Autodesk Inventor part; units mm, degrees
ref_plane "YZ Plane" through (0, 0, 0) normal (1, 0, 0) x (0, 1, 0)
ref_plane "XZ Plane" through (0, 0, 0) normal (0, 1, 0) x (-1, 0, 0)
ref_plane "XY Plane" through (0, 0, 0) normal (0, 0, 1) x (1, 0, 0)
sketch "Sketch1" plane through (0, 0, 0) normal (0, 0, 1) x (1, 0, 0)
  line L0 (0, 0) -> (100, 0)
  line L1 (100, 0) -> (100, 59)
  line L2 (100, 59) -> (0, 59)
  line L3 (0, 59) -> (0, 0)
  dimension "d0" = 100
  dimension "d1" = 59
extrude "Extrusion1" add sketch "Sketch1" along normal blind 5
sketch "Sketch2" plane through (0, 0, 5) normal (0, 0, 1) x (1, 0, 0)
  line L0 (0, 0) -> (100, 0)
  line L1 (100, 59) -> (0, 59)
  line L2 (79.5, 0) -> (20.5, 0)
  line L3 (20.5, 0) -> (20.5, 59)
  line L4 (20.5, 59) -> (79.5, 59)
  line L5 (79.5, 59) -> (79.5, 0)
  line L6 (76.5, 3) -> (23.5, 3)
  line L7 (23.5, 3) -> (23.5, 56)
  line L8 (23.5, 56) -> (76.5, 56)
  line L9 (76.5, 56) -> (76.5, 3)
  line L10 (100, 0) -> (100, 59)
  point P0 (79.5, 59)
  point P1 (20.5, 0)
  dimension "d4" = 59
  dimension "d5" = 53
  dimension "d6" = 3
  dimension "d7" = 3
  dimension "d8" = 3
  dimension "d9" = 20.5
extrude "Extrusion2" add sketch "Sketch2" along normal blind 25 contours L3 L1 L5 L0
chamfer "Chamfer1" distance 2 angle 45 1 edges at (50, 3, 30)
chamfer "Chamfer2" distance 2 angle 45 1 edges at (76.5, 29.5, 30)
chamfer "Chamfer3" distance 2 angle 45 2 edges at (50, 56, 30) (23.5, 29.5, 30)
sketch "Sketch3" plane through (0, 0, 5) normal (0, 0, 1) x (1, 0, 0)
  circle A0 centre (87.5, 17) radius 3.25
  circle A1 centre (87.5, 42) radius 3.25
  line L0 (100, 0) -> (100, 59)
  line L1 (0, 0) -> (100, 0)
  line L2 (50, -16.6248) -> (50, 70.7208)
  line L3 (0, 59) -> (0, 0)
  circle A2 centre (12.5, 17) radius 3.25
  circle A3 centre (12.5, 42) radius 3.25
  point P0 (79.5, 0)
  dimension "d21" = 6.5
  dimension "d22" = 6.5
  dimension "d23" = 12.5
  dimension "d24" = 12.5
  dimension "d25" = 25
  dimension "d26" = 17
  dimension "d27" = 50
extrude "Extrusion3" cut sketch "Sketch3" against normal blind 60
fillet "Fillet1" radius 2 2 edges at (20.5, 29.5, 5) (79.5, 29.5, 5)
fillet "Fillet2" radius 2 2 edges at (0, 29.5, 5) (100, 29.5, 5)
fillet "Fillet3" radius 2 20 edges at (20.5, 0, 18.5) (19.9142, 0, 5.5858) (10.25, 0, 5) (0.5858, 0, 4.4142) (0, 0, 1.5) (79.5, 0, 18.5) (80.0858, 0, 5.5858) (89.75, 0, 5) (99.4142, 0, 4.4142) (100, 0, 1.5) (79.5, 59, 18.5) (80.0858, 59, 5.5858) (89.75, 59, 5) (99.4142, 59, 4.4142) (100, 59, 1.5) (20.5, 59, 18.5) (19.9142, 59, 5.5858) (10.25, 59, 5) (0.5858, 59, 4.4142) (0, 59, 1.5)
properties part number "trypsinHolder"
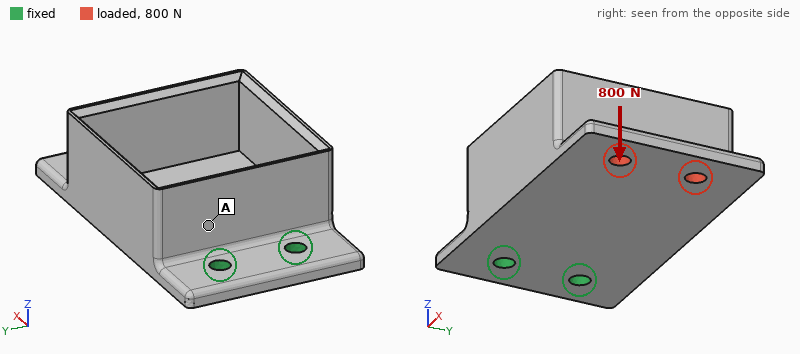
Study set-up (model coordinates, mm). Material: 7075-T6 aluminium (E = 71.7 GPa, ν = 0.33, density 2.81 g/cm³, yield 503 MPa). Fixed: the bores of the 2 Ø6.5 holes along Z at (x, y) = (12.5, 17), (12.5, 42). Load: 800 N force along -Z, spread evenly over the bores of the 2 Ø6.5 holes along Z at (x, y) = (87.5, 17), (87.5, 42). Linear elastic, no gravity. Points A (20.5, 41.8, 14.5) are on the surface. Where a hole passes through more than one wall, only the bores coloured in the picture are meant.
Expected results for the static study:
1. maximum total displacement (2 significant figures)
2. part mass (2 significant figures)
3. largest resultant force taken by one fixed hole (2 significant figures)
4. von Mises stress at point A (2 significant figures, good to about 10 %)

1.4 mm
130 g
470 N
37 MPa
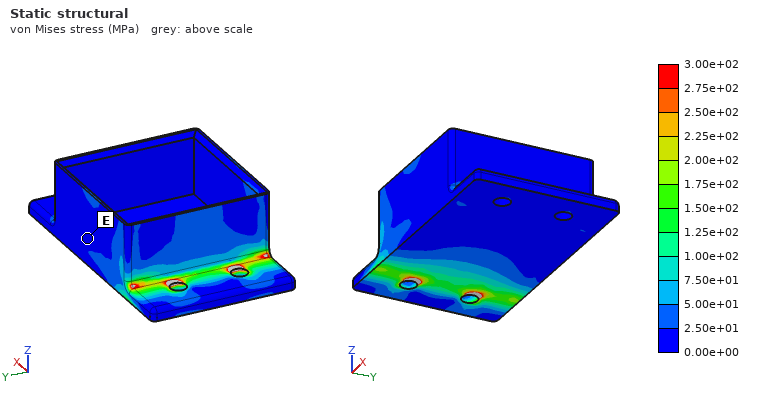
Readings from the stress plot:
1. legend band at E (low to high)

0.00e+00 to 2.50e+01 MPa
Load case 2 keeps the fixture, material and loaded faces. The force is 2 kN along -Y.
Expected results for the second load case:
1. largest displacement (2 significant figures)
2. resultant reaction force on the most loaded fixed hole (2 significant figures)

0.12 mm
5.1 kN
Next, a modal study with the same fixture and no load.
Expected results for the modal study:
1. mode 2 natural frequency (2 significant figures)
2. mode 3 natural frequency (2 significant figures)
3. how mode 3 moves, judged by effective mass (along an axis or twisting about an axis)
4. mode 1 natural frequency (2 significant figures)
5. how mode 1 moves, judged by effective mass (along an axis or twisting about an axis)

1400 Hz
3300 Hz
along Y
630 Hz
along Z
